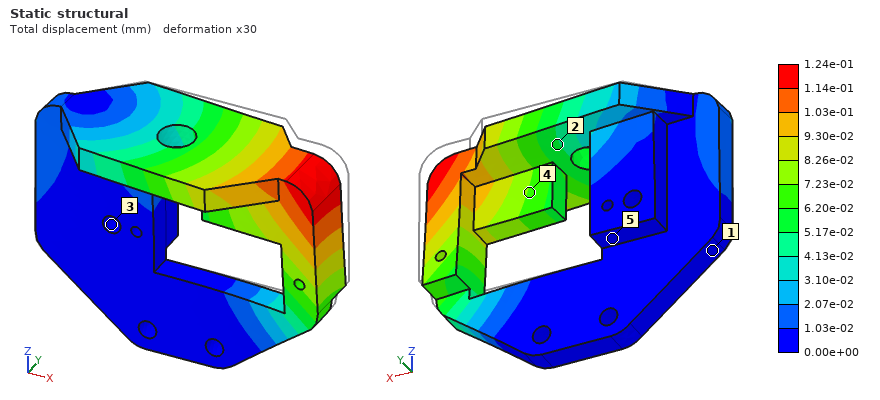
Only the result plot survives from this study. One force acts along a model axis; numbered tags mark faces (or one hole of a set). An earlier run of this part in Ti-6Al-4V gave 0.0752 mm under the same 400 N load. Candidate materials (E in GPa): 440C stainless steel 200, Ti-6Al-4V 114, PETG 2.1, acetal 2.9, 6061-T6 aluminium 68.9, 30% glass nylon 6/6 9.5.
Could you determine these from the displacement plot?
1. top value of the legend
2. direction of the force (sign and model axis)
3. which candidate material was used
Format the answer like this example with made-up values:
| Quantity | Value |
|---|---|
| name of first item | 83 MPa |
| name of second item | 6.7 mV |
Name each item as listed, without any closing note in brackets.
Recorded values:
| Quantity | Value |
|---|---|
| top value of the legend | 1.24e-01 mm |
| direction of the force | -Y |
| which candidate material was used | 6061-T6 aluminium |
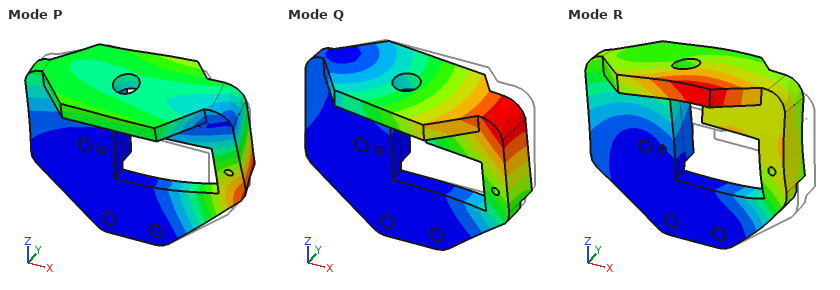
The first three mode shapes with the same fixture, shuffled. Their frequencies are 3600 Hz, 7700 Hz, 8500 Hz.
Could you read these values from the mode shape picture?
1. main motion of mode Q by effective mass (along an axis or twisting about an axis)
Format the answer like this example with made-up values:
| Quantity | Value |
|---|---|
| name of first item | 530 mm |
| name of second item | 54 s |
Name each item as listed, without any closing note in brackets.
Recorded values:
| Quantity | Value |
|---|---|
| main motion of mode Q by effective mass | along Y |
